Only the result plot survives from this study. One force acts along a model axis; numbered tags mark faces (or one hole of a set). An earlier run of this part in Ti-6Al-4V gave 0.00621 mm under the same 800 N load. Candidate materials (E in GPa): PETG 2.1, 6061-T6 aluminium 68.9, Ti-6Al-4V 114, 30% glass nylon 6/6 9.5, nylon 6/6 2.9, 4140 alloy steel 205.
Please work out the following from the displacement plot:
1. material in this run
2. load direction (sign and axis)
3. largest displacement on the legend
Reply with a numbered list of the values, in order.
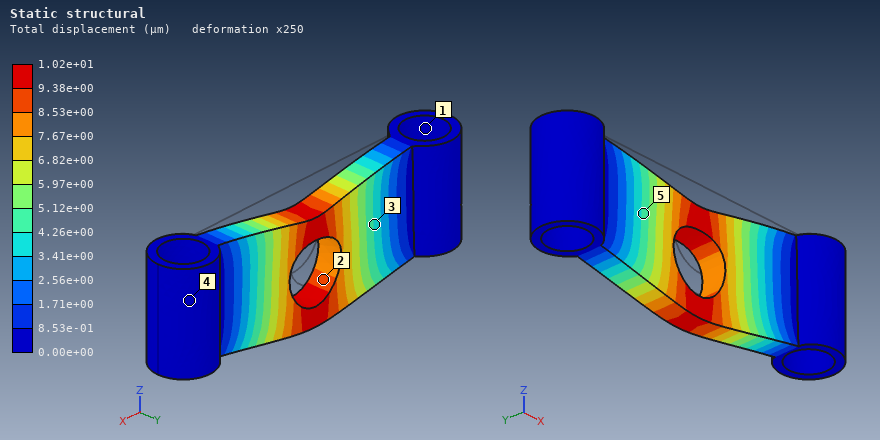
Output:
1. 6061-T6 aluminium
2. -Z
3. 1.02e+01 µm
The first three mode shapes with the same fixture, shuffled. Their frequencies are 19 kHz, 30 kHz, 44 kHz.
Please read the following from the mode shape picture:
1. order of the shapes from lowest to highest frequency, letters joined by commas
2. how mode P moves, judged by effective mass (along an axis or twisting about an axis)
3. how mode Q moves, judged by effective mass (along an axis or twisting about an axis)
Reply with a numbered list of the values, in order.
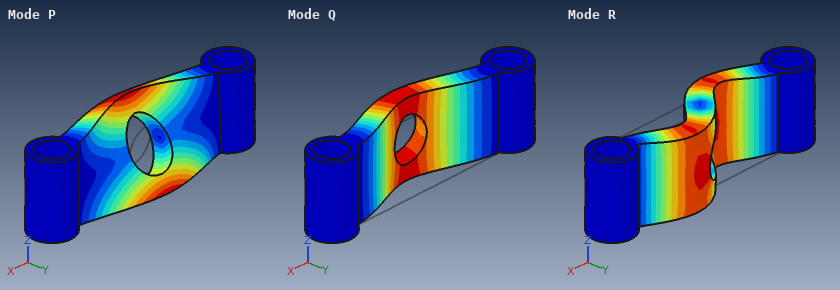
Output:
1. Q, P, R
2. twisting about X
3. along Y
